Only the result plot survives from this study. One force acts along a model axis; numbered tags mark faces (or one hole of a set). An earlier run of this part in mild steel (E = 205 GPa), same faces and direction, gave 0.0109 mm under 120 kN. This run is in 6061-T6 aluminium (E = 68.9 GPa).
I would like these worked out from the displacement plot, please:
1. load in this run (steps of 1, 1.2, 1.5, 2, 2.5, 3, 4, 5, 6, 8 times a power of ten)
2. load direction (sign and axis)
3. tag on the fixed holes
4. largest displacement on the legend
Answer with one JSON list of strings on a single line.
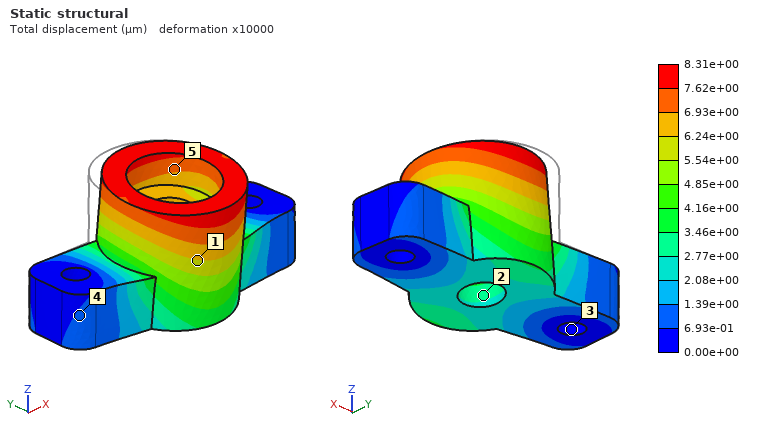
["30 kN", "-Y", "3", "8.31e+00 µm"]
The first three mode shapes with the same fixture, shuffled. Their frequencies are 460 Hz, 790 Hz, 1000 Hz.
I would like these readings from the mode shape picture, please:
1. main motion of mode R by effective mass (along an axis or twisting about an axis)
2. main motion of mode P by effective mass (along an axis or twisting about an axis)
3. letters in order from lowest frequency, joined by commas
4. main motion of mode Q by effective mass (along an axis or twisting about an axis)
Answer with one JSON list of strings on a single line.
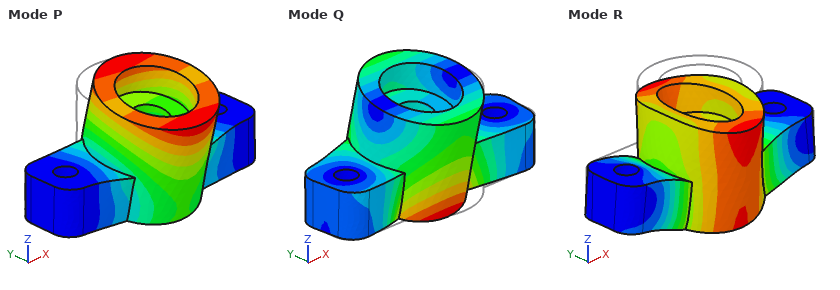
["along Z", "along Y", "P, R, Q", "along Y"]
